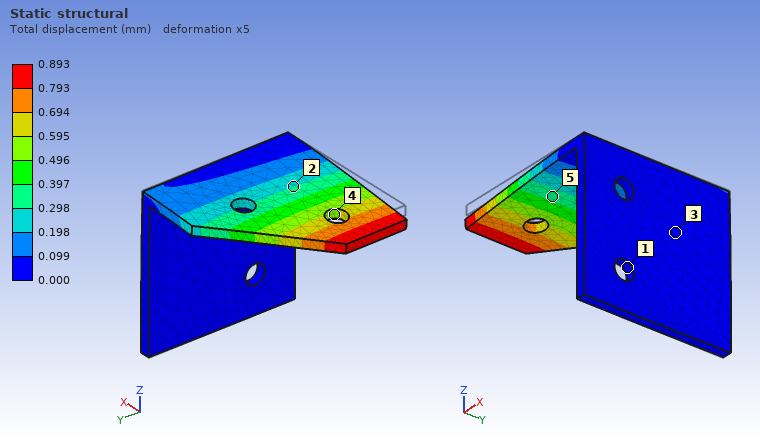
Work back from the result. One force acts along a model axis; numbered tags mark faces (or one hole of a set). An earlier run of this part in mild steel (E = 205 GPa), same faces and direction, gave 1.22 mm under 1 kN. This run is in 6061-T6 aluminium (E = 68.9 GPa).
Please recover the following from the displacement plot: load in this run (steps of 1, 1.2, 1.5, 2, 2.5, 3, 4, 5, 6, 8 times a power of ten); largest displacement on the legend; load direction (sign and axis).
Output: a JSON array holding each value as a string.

["250 N", "0.893 mm", "-Z"]
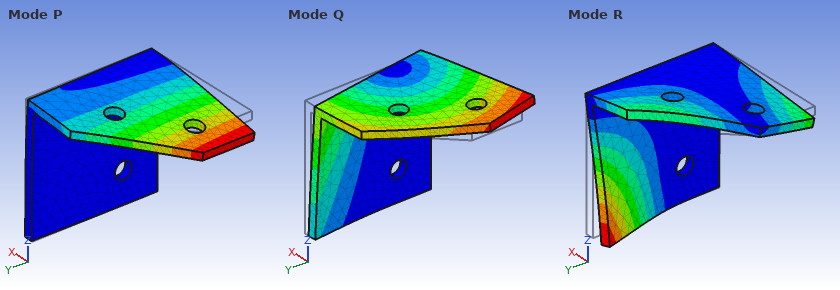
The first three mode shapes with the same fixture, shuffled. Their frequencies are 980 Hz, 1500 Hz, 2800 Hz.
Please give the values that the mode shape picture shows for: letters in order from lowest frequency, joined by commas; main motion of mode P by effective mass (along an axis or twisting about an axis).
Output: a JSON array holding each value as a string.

["P, Q, R", "along Z"]
